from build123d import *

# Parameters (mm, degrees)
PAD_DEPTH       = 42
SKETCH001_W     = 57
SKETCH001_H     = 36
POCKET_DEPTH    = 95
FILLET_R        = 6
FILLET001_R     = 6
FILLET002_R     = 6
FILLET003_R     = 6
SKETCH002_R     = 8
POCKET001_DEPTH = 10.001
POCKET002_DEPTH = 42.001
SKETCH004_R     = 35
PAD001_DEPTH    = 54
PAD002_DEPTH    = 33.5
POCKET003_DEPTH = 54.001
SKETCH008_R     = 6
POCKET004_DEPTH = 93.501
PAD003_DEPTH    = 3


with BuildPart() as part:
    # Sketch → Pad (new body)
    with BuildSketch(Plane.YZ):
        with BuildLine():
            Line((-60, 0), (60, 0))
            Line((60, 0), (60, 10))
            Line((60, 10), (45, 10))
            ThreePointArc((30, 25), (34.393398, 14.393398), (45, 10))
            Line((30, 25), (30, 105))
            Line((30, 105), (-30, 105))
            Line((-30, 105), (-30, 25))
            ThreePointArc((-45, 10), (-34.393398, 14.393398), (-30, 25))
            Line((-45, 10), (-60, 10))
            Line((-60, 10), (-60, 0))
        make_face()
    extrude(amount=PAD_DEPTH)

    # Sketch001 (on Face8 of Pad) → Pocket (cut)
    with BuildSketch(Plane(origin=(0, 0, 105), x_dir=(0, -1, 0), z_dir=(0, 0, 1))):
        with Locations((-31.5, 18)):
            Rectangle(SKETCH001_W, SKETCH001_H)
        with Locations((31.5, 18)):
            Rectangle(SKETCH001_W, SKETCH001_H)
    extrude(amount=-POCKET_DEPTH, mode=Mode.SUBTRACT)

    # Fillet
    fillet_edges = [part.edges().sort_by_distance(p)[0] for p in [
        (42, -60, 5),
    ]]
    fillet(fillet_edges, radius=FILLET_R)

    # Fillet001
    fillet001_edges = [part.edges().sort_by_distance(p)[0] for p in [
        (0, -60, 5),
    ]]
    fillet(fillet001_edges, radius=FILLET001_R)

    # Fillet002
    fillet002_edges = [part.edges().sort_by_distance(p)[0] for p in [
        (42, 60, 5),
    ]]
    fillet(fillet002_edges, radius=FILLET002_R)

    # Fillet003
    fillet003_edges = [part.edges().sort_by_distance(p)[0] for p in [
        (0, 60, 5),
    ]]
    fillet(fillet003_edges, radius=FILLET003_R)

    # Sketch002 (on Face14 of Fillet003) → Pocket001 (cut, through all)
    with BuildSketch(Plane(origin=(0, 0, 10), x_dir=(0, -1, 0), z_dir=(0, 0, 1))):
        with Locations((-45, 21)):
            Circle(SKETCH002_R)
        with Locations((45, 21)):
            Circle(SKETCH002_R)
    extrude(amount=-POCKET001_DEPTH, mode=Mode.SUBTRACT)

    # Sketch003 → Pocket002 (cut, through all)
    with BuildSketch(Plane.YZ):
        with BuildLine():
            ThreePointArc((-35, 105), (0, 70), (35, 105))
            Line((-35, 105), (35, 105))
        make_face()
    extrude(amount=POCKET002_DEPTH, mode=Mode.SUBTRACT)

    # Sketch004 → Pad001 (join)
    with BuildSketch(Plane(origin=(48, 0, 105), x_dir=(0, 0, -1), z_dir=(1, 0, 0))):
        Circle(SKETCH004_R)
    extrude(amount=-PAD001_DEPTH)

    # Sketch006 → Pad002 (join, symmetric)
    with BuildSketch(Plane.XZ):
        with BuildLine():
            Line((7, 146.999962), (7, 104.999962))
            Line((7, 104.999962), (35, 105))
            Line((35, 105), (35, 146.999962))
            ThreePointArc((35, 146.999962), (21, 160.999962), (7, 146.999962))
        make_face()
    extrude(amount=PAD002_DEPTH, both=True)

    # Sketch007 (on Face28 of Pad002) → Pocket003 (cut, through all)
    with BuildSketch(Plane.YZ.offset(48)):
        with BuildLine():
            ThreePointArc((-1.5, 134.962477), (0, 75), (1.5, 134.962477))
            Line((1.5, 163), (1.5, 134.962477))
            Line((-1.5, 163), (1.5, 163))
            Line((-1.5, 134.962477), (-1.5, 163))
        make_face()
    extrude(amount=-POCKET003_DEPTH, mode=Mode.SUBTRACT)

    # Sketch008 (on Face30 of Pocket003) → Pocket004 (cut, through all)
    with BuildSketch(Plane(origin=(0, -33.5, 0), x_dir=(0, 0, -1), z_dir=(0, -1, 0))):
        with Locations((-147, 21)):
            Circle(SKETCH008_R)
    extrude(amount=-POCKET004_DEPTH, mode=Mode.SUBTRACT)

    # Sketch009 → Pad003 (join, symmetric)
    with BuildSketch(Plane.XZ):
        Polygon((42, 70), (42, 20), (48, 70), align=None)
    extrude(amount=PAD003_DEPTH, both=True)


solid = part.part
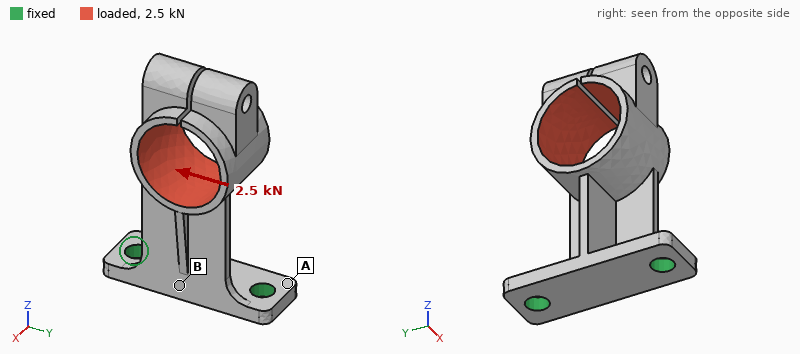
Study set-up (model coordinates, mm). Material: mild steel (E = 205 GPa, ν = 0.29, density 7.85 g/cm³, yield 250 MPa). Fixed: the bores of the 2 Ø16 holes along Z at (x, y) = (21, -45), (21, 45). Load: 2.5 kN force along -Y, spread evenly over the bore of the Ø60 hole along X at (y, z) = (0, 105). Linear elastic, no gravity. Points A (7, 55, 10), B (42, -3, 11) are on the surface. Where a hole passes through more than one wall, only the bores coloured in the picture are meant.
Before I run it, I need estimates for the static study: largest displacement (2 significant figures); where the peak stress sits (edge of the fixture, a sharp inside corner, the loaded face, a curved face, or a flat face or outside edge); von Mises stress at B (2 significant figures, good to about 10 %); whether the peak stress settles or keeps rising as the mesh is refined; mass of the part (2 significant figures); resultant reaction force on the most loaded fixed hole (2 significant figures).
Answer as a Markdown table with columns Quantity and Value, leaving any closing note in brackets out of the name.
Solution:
| Quantity | Value |
|---|---|
| largest displacement | 0.73 mm |
| where the peak stress sits | a sharp inside corner |
| von Mises stress at B | 48 MPa |
| whether the peak stress settles or keeps rising as the mesh is refined | keeps rising |
| mass of the part | 1.4 kg |
| resultant reaction force on the most loaded fixed hole | 3.7 kN |
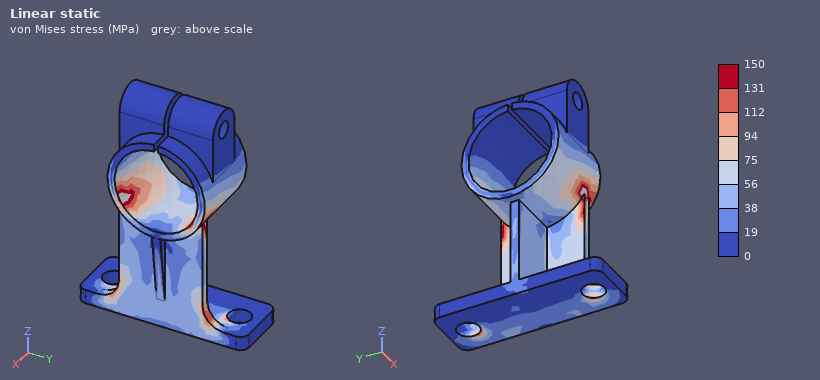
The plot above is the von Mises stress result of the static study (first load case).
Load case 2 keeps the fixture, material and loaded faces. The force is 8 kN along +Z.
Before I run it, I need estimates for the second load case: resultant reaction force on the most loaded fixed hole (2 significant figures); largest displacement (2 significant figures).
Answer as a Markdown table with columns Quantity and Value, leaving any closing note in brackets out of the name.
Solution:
| Quantity | Value |
|---|---|
| resultant reaction force on the most loaded fixed hole | 4.1 kN |
| largest displacement | 0.47 mm |
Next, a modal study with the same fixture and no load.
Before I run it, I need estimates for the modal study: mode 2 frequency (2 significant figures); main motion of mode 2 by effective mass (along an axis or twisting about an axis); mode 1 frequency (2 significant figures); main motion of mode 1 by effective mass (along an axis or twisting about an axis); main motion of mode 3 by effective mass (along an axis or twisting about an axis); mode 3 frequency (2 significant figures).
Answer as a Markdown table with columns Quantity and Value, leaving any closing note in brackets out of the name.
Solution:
| Quantity | Value |
|---|---|
| mode 2 frequency | 330 Hz |
| main motion of mode 2 by effective mass | along X |
| mode 1 frequency | 320 Hz |
| main motion of mode 1 by effective mass | along Y |
| main motion of mode 3 by effective mass | along X |
| mode 3 frequency | 410 Hz |
